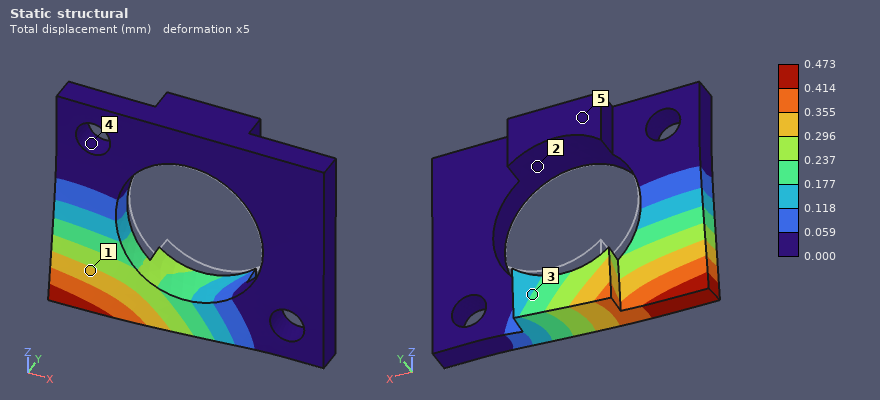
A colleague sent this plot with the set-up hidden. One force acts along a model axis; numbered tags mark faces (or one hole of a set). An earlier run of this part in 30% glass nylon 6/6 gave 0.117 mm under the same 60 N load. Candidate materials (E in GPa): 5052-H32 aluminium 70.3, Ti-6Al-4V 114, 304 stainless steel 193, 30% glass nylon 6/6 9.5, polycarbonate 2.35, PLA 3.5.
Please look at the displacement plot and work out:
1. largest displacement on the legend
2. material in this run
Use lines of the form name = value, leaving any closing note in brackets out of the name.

largest displacement on the legend = 0.473 mm
material in this run = polycarbonate
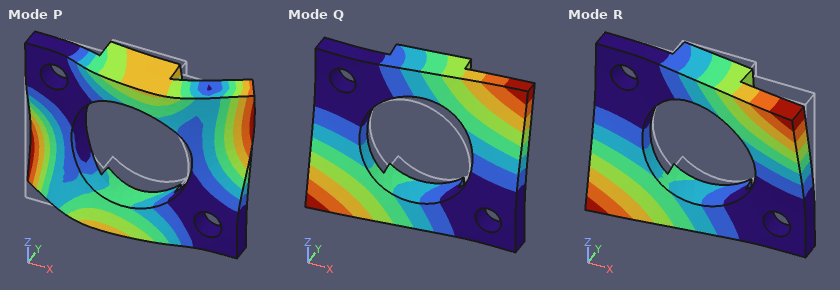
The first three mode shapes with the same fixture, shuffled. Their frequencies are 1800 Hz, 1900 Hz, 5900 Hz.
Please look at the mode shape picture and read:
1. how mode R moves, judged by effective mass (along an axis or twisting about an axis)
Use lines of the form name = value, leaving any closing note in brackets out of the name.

how mode R moves, judged by effective mass = along Y
